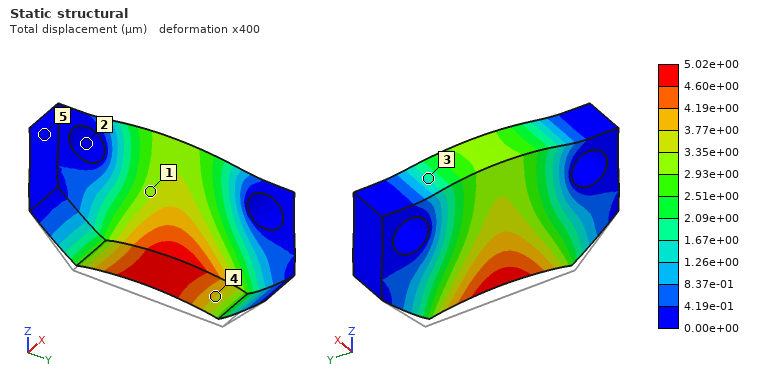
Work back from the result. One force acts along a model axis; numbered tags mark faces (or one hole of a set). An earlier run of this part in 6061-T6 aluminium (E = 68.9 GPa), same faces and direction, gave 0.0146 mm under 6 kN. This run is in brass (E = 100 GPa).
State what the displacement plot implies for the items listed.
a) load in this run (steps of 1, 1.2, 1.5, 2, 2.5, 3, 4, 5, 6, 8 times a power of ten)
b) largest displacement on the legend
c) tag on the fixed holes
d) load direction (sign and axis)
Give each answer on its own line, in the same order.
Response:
3 kN
5.02e+00 µm
2
+Z
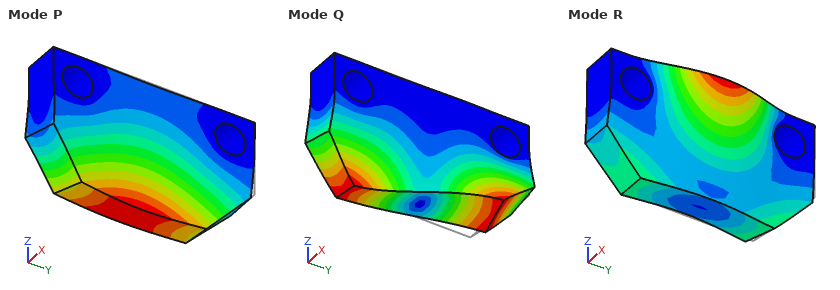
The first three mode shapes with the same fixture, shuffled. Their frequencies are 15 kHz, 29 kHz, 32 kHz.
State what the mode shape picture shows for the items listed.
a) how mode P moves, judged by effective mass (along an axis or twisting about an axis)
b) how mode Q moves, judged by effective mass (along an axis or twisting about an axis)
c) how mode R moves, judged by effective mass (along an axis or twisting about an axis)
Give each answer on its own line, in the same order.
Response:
along X
twisting about Z
along X
